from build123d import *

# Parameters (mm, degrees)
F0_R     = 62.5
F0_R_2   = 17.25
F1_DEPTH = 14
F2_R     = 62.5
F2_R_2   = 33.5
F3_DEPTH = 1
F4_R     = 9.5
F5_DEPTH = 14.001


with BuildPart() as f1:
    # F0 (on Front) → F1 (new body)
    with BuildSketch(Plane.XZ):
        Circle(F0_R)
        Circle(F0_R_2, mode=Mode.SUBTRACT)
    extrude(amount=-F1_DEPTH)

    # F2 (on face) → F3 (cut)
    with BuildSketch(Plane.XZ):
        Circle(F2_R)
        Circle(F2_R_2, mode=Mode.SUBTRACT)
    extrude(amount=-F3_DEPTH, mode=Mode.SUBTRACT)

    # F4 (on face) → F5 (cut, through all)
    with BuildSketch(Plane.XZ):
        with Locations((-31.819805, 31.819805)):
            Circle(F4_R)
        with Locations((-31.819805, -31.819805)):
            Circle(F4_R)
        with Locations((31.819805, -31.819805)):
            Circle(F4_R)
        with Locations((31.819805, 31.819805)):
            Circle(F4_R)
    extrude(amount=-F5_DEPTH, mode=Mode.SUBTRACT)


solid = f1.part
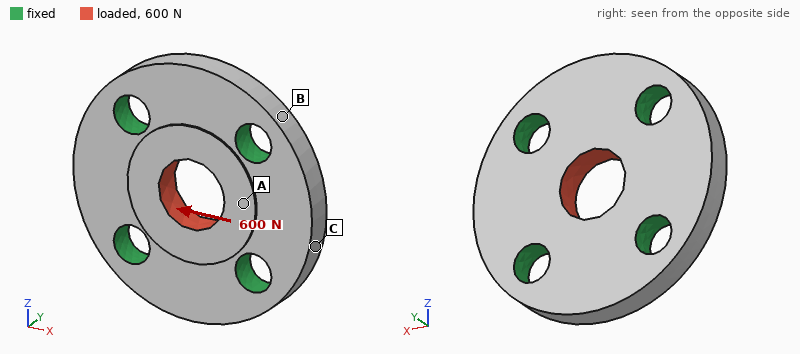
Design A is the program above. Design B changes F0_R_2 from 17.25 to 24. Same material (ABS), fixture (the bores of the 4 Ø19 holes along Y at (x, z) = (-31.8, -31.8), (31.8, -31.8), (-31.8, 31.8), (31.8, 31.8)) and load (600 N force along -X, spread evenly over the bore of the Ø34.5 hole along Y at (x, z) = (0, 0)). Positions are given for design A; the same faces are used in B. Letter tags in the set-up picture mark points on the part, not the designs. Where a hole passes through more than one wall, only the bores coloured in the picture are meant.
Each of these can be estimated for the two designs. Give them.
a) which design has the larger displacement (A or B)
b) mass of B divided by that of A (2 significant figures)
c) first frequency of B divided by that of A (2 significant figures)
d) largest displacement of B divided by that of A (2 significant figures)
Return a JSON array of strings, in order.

["A", "0.91", "0.99", "0.89"]
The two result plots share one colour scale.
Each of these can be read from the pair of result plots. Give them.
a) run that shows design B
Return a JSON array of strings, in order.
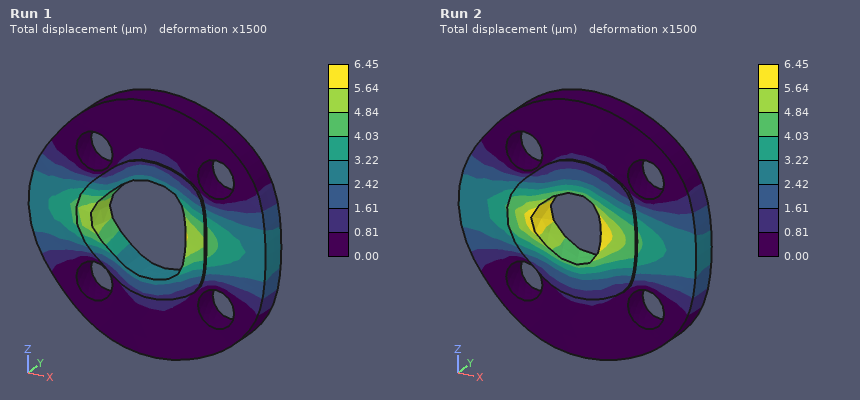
["Run 1"]
